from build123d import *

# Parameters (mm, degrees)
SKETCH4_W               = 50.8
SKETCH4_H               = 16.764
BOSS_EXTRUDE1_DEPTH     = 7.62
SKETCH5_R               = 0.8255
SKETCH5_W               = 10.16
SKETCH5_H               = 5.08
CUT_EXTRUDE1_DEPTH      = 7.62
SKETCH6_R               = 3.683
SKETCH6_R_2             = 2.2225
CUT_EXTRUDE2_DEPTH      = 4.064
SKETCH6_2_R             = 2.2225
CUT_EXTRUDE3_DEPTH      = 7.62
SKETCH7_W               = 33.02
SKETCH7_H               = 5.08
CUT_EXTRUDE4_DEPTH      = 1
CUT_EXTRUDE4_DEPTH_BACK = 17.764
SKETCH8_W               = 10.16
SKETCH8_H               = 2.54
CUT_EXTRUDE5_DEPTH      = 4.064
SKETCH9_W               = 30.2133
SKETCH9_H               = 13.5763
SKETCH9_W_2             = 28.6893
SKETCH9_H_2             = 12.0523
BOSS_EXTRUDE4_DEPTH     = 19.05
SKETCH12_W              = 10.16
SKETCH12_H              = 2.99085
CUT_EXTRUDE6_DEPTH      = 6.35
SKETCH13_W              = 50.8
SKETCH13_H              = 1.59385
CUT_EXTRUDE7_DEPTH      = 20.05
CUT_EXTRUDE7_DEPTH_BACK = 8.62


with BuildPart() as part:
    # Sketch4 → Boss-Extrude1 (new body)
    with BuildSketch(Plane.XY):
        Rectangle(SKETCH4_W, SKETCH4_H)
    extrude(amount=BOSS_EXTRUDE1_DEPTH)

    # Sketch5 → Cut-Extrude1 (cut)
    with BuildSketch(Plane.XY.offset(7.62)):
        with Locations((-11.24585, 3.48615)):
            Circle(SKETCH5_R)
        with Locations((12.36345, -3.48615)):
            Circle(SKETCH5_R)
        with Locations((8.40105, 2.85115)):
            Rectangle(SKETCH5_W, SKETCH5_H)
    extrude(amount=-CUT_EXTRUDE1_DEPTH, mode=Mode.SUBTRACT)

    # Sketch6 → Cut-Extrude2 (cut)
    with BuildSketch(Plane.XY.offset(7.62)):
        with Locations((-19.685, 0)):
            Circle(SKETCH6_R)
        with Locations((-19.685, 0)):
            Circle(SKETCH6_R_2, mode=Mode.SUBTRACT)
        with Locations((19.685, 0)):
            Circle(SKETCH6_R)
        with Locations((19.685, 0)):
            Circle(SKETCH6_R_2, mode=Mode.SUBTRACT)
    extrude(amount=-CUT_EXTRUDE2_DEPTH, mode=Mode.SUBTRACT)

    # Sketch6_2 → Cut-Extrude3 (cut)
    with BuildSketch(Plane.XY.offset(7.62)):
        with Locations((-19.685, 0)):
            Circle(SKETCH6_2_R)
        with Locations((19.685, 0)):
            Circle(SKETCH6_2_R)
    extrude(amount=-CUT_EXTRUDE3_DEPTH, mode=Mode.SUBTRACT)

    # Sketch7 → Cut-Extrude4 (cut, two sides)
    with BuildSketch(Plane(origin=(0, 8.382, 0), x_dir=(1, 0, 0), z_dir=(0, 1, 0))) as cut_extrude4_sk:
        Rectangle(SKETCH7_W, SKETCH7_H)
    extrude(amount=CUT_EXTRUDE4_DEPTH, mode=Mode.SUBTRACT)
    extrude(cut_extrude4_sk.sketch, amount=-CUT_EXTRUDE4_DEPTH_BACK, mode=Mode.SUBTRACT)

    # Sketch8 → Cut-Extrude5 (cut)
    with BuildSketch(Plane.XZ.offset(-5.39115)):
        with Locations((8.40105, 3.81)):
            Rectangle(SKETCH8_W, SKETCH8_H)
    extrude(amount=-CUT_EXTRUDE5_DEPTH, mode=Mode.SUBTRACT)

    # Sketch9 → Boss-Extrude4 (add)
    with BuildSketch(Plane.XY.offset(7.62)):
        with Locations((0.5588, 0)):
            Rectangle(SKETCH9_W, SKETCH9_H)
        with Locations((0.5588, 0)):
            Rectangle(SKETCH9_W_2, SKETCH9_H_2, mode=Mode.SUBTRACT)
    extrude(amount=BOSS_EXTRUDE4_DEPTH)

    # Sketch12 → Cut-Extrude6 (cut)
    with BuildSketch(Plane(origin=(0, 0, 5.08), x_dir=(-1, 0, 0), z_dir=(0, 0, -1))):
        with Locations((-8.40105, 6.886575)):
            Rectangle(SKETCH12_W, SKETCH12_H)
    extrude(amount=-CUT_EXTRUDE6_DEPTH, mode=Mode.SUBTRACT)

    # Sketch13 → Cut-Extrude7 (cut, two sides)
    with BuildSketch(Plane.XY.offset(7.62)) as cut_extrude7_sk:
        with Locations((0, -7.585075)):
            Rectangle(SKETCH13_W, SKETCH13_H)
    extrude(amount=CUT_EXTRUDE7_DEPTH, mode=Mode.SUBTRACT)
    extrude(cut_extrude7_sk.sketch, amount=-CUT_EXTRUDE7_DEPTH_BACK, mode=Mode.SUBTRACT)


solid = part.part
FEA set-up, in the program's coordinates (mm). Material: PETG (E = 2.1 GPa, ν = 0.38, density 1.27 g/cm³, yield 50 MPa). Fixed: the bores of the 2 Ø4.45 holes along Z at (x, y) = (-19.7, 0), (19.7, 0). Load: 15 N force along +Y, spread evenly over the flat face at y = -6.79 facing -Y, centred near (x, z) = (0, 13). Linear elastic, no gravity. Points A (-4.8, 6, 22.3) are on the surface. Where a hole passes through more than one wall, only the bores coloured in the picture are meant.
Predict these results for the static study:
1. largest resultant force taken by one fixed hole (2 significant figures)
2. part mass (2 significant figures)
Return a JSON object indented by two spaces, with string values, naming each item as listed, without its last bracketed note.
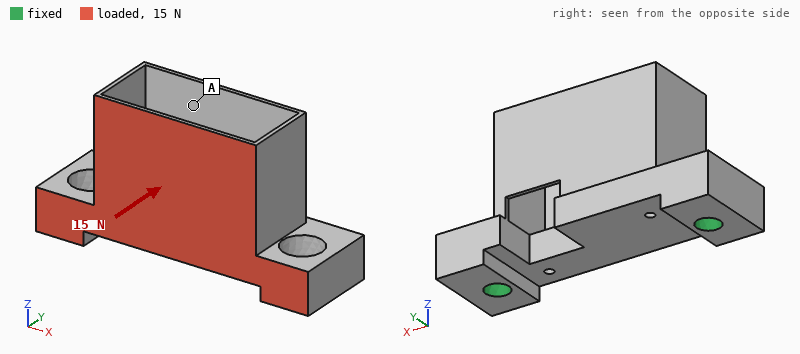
{
  "largest resultant force taken by one fixed hole": "7.6 N",
  "part mass": "6.2 g"
}
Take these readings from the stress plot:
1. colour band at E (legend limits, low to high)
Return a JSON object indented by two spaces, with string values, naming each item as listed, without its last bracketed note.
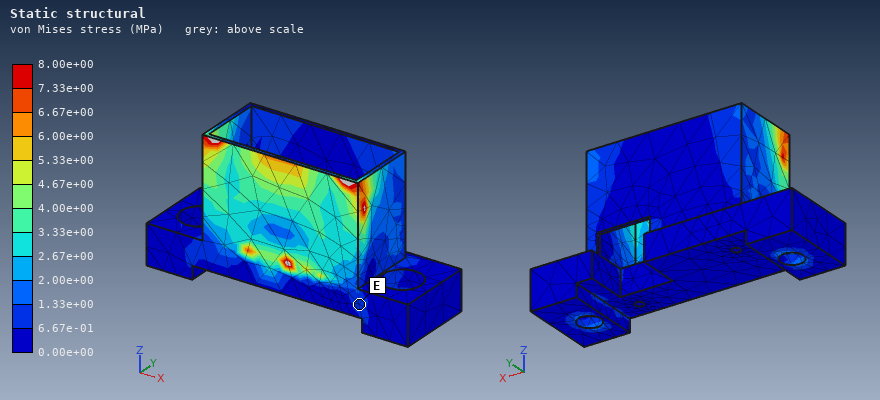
{
  "colour band at E": "6.67e-01 to 1.33e+00 MPa"
}
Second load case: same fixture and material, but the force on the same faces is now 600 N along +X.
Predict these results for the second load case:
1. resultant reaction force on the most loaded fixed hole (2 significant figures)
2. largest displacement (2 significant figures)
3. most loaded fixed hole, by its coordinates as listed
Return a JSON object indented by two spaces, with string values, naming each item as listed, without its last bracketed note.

{
  "resultant reaction force on the most loaded fixed hole": "380 N",
  "largest displacement": "0.56 mm",
  "most loaded fixed hole, by its coordinates as listed": "(-19.7, 0)"
}
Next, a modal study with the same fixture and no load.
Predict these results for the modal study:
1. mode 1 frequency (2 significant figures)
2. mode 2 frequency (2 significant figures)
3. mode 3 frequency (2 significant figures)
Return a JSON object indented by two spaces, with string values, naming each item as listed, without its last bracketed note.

{
  "mode 1 frequency": "1100 Hz",
  "mode 2 frequency": "1200 Hz",
  "mode 3 frequency": "2500 Hz"
}
